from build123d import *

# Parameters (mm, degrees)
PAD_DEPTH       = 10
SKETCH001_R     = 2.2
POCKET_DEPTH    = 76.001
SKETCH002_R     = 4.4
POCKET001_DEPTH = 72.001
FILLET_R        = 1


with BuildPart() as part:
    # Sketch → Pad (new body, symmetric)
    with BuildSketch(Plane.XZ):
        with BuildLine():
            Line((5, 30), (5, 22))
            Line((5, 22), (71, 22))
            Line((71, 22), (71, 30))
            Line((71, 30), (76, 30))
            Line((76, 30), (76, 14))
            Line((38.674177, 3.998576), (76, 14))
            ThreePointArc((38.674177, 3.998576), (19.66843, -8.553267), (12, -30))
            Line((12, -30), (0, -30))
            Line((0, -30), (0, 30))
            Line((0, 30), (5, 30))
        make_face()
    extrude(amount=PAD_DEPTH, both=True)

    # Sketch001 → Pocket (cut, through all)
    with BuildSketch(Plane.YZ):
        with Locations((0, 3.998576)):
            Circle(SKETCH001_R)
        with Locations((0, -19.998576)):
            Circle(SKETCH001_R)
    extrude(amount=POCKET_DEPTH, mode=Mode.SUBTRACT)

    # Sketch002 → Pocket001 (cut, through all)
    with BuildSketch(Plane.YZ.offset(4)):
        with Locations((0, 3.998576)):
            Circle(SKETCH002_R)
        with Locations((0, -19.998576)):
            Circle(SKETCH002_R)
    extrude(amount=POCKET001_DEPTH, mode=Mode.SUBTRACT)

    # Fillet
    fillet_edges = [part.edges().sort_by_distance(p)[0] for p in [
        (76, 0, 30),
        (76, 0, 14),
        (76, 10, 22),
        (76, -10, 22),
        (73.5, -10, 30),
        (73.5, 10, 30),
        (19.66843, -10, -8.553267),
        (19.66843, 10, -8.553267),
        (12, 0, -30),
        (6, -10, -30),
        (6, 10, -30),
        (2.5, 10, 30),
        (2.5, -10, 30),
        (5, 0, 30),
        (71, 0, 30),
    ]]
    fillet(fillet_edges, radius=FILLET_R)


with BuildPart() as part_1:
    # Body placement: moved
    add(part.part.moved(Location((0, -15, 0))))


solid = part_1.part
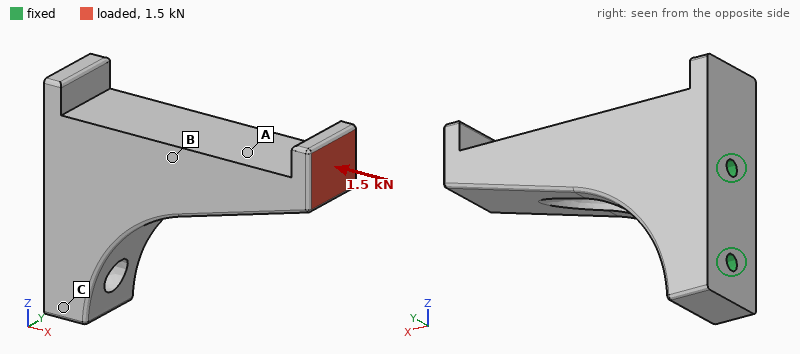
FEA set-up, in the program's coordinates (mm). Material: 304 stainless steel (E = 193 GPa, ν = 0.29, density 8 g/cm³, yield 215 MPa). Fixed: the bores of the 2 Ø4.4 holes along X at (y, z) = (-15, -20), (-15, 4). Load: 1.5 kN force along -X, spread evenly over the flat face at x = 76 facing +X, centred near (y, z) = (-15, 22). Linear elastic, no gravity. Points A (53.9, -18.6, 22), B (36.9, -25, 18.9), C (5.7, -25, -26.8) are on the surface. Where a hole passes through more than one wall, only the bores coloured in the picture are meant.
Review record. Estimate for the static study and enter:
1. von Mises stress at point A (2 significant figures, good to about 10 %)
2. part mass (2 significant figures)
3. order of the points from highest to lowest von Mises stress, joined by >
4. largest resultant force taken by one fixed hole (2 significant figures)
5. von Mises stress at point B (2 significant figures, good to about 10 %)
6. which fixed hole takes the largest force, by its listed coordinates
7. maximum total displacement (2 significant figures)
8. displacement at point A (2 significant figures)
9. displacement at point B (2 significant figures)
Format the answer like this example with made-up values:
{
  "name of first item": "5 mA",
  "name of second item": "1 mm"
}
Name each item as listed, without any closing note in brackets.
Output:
{
  "von Mises stress at point A": "22 MPa",
  "part mass": "280 g",
  "order of the points from highest to lowest von Mises stress, joined by >": "A > B > C",
  "largest resultant force taken by one fixed hole": "2.5 kN",
  "von Mises stress at point B": "12 MPa",
  "which fixed hole takes the largest force, by its listed coordinates": "(-15, 4)",
  "maximum total displacement": "38 µm",
  "displacement at point A": "18 µm",
  "displacement at point B": "11 µm"
}
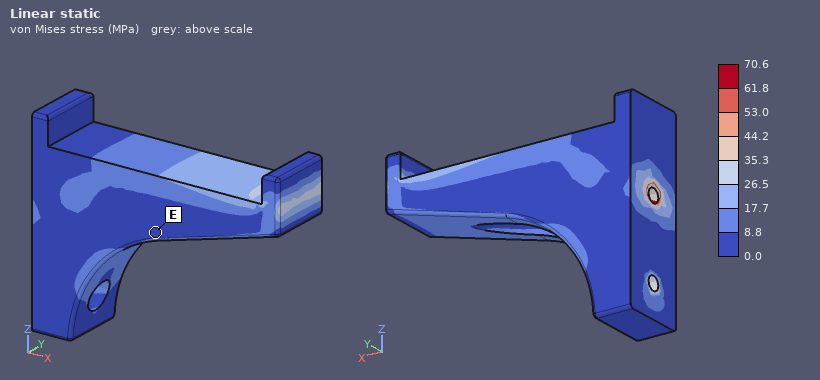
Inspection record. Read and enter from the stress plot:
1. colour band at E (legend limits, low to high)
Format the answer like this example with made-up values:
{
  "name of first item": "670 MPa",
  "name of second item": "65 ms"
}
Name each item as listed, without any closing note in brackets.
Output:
{
  "colour band at E": "0.0 to 8.8 MPa"
}
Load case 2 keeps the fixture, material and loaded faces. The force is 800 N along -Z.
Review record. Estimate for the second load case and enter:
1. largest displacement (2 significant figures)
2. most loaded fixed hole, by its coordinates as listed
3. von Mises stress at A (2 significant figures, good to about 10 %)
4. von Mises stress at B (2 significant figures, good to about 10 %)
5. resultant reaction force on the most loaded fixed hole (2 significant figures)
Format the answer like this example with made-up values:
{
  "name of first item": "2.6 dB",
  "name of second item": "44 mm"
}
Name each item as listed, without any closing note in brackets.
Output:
{
  "largest displacement": "64 µm",
  "most loaded fixed hole, by its coordinates as listed": "(-15, -20)",
  "von Mises stress at A": "29 MPa",
  "von Mises stress at B": "19 MPa",
  "resultant reaction force on the most loaded fixed hole": "2.6 kN"
}
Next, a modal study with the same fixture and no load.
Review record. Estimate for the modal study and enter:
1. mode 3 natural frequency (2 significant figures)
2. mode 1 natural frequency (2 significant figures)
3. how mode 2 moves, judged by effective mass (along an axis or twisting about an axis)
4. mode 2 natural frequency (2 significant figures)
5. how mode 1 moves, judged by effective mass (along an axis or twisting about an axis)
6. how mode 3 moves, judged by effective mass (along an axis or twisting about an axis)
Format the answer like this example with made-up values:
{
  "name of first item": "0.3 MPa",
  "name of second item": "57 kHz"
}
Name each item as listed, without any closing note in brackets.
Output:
{
  "mode 3 natural frequency": "9000 Hz",
  "mode 1 natural frequency": "1300 Hz",
  "how mode 2 moves, judged by effective mass": "along Z",
  "mode 2 natural frequency": "2900 Hz",
  "how mode 1 moves, judged by effective mass": "along Y",
  "how mode 3 moves, judged by effective mass": "along X"
}
